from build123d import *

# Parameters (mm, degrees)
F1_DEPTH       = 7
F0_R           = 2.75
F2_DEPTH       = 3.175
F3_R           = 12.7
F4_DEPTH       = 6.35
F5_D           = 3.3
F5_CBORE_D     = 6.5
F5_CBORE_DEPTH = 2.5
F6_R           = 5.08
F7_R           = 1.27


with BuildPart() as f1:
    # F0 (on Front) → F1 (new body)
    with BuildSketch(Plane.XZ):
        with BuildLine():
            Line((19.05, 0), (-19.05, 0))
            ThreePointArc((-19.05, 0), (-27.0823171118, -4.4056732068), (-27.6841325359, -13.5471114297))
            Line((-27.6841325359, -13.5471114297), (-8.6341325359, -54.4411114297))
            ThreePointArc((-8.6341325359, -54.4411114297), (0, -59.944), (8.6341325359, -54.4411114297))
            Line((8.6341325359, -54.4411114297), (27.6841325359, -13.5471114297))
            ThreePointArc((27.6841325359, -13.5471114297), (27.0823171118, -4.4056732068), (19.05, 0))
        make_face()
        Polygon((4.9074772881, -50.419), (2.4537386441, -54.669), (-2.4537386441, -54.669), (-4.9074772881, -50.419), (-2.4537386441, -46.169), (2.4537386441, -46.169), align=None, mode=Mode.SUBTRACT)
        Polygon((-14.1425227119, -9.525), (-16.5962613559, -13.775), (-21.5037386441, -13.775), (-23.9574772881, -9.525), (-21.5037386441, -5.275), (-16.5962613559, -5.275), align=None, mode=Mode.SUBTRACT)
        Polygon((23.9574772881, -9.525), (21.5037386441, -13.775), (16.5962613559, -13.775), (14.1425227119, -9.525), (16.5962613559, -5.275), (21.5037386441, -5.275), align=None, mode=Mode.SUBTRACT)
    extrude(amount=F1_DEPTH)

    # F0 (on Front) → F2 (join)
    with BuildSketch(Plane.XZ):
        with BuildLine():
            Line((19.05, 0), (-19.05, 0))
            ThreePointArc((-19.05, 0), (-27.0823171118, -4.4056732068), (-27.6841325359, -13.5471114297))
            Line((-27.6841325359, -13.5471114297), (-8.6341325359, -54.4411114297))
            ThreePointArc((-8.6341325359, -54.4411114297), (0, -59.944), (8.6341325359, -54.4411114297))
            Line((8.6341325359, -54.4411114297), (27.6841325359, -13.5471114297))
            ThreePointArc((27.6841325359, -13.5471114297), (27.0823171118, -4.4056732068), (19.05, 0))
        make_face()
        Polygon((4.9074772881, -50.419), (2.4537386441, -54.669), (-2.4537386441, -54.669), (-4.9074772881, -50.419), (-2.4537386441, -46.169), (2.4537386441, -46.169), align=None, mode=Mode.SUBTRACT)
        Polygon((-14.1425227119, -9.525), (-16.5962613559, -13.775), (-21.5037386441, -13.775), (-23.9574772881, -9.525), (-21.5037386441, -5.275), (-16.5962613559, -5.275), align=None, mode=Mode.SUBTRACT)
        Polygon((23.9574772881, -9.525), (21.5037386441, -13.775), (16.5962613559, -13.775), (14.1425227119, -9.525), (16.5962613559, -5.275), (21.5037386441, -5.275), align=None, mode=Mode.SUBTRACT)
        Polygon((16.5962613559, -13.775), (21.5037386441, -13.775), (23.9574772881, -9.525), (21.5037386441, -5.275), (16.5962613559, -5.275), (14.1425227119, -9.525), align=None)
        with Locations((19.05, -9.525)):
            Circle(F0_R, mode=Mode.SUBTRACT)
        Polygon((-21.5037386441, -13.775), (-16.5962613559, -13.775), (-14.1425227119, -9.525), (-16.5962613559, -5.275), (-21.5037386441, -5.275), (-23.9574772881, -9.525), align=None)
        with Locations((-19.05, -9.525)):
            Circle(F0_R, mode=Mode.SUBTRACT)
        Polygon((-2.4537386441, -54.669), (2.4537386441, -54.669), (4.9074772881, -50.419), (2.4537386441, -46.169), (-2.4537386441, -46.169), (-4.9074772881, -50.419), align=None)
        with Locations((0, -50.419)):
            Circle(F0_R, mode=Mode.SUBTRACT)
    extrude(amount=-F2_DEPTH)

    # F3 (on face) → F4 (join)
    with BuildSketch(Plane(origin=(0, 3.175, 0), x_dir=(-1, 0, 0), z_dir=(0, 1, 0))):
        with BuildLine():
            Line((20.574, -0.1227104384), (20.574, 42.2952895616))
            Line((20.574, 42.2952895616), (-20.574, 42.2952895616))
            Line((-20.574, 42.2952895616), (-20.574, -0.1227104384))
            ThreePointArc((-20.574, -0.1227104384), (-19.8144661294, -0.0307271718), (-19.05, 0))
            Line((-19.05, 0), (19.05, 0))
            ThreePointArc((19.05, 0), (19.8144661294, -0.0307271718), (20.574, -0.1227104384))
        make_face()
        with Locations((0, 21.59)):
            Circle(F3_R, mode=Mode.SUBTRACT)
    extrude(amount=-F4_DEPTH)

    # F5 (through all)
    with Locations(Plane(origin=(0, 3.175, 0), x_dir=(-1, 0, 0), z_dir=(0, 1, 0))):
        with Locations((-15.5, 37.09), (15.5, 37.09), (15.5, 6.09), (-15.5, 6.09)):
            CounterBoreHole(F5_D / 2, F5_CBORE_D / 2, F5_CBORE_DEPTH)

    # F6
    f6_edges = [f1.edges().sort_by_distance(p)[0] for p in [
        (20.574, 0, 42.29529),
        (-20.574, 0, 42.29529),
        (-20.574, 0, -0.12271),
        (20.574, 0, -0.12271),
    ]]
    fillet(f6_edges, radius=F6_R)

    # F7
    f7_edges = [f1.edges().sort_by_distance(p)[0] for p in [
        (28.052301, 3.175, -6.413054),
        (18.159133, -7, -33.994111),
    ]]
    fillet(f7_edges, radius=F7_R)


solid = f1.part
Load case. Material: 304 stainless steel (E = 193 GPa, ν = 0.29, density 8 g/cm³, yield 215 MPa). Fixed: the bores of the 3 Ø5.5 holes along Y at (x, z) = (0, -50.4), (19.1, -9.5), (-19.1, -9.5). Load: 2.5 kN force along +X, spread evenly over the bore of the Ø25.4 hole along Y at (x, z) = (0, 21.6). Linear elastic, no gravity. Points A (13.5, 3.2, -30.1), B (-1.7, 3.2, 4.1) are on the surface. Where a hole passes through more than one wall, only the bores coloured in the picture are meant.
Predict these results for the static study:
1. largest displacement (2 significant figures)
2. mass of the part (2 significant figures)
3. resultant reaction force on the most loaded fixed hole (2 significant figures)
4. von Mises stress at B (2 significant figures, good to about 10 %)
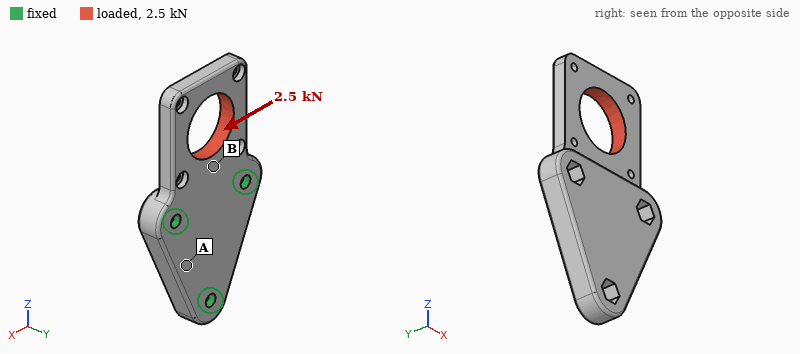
29 µm
230 g
2.2 kN
38 MPa
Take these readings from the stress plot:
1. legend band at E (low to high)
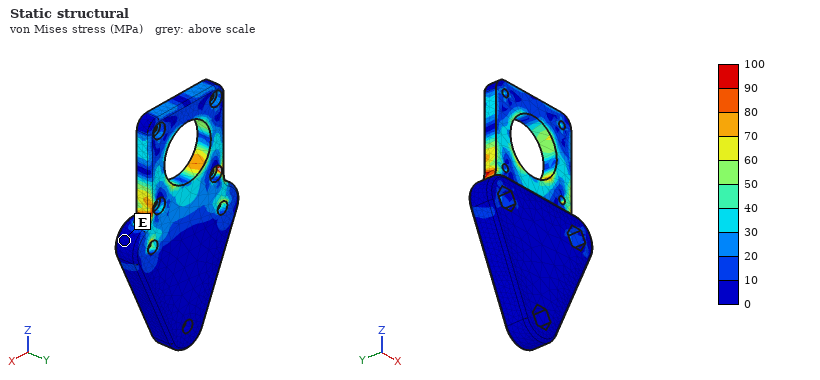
0 to 10 MPa
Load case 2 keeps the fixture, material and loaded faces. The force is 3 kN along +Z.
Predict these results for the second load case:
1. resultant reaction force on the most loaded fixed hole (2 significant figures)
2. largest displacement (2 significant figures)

1.2 kN
8.4 µm
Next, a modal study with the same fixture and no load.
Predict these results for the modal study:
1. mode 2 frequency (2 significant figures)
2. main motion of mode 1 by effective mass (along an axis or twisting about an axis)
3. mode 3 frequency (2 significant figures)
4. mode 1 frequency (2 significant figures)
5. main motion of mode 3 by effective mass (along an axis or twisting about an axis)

4800 Hz
along Y
7000 Hz
2000 Hz
along X
